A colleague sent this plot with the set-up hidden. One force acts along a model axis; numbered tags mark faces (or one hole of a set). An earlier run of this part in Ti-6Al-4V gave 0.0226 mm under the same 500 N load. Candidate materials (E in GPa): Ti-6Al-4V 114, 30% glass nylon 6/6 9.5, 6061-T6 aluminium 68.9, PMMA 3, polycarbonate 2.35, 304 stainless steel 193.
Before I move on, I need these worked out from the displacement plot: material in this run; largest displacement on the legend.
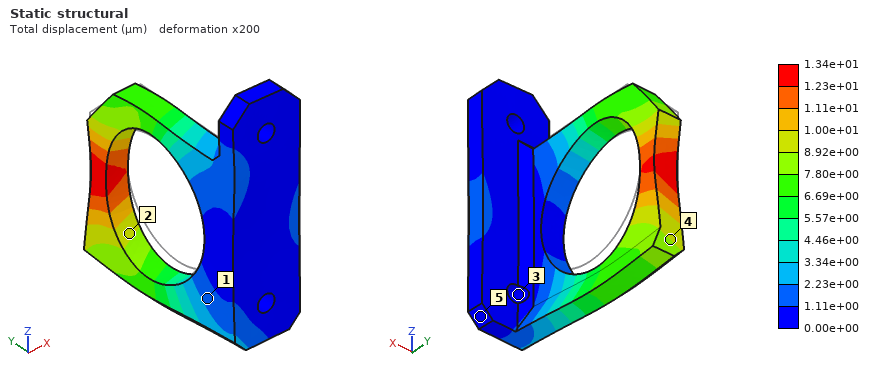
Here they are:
304 stainless steel
1.34e+01 µm
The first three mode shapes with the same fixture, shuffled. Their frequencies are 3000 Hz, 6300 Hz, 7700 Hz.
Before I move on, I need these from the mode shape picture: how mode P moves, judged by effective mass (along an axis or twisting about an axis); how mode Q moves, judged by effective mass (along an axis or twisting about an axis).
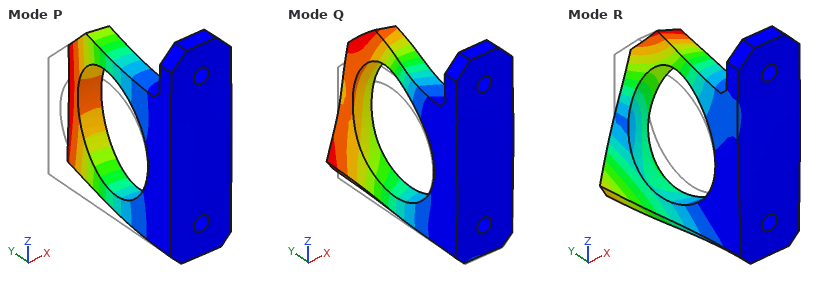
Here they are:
along X
along Z
